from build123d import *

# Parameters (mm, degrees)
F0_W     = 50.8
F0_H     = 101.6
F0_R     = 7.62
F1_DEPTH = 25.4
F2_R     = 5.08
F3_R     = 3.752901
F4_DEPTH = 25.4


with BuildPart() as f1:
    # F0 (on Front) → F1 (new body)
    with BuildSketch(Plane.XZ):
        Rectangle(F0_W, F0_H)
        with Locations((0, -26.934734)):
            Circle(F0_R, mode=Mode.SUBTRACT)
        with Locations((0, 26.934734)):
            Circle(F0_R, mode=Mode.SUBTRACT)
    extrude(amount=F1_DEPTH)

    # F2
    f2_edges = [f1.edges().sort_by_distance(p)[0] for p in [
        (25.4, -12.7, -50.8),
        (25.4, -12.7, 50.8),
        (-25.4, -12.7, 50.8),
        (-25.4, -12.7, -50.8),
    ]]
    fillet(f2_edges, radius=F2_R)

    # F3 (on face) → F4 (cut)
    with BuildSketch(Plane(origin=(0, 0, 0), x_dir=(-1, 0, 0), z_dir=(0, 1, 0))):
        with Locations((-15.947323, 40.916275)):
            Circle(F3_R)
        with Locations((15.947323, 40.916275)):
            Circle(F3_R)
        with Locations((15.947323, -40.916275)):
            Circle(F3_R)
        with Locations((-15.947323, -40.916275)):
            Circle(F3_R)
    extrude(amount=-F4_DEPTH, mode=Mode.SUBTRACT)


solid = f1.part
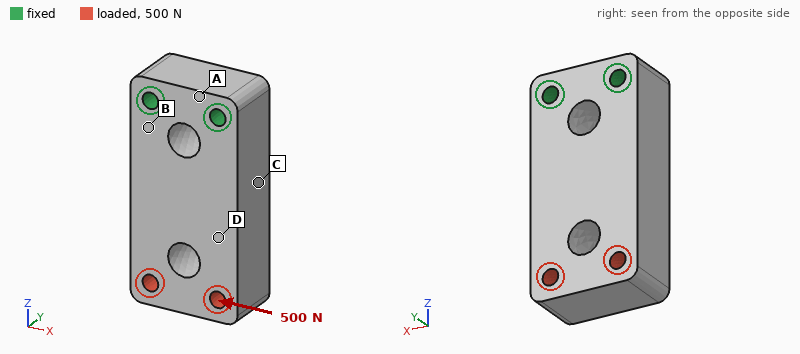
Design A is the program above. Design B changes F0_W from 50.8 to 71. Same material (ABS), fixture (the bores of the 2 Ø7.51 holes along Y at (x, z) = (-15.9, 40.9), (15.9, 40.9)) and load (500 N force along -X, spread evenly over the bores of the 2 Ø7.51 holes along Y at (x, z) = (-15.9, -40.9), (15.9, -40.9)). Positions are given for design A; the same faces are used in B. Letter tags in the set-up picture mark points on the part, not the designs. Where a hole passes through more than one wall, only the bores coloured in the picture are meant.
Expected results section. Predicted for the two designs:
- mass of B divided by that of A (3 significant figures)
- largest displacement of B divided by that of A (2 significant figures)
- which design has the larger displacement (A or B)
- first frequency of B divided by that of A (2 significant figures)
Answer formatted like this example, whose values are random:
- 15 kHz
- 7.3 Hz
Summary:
- 1.45
- 0.72
- A
- 0.95
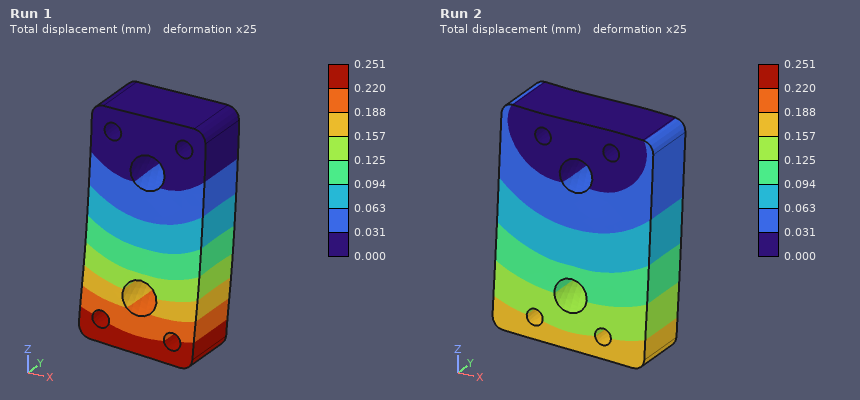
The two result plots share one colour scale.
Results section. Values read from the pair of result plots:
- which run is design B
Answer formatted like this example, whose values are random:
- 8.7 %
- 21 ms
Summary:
- Run 2
